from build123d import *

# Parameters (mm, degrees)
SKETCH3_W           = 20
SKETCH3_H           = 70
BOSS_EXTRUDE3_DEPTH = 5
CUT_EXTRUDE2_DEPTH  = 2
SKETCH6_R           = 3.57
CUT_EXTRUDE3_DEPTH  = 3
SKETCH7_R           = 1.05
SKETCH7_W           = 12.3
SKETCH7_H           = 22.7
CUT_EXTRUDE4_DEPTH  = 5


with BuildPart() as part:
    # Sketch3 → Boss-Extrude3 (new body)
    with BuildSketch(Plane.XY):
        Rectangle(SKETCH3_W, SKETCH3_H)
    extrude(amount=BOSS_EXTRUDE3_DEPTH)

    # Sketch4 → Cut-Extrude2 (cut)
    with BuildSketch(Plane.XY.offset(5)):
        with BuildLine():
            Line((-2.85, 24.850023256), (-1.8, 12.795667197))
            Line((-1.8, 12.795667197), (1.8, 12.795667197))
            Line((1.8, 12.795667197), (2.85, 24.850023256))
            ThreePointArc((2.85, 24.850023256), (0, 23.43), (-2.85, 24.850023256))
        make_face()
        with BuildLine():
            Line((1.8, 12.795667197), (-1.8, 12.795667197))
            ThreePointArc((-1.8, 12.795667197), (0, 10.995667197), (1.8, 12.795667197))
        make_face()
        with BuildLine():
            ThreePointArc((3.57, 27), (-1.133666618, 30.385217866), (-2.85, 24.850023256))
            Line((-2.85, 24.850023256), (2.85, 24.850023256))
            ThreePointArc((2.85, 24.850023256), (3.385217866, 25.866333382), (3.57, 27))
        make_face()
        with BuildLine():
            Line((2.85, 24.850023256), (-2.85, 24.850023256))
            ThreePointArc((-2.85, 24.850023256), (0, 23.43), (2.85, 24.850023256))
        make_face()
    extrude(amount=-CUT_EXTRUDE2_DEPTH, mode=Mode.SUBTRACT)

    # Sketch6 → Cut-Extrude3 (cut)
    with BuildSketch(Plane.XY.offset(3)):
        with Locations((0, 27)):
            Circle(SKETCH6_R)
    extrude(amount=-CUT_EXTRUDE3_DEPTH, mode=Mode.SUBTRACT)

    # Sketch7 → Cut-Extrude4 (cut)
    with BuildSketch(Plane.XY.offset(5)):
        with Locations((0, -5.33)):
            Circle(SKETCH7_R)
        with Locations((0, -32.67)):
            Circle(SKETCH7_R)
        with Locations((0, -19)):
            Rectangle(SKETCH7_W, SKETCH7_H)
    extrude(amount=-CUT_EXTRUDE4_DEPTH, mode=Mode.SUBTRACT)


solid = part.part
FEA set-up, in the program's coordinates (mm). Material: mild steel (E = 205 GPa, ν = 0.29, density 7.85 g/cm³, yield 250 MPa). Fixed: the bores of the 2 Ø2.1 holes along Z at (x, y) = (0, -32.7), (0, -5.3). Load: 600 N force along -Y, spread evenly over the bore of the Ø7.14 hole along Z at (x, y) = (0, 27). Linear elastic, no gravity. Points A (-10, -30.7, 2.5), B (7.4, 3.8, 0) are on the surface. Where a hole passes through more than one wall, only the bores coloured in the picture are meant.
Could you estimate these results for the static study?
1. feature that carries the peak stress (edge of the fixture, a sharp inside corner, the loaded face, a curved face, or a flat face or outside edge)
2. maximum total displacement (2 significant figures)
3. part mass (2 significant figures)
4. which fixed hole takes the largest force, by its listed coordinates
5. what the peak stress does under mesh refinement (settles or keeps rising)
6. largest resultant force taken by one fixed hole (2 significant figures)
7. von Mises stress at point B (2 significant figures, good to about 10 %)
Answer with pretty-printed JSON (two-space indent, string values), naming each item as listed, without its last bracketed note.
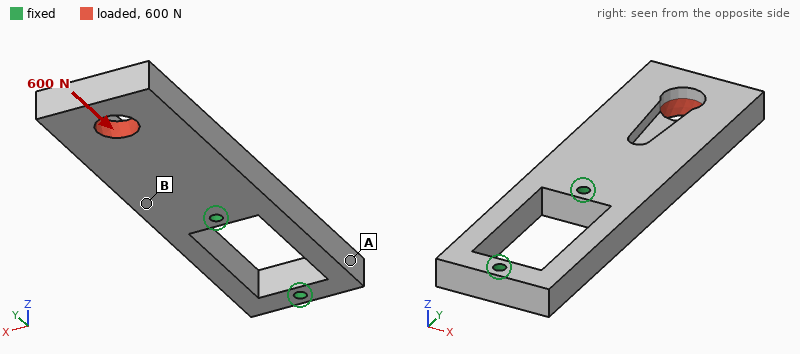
{
  "feature that carries the peak stress": "edge of the fixture",
  "maximum total displacement": "13 µm",
  "part mass": "41 g",
  "which fixed hole takes the largest force, by its listed coordinates": "(0, -5.3)",
  "what the peak stress does under mesh refinement": "keeps rising",
  "largest resultant force taken by one fixed hole": "550 N",
  "von Mises stress at point B": "12 MPa"
}
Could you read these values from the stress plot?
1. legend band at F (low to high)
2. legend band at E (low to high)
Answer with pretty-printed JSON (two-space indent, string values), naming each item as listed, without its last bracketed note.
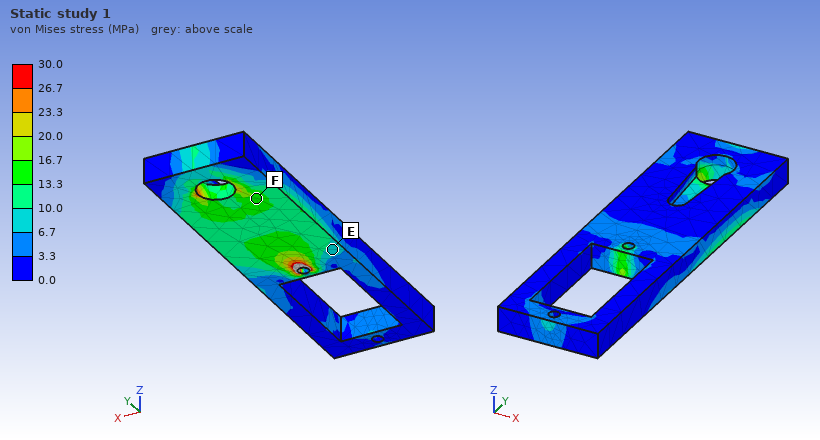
{
  "legend band at F": "13.3 to 16.7 MPa",
  "legend band at E": "6.7 to 10.0 MPa"
}
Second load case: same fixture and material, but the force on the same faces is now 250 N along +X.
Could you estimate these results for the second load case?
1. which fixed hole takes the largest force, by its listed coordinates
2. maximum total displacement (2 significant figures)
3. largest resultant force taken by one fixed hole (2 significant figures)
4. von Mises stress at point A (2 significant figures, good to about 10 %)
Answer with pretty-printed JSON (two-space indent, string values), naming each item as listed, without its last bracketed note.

{
  "which fixed hole takes the largest force, by its listed coordinates": "(0, -5.3)",
  "maximum total displacement": "34 µm",
  "largest resultant force taken by one fixed hole": "340 N",
  "von Mises stress at point A": "22 MPa"
}
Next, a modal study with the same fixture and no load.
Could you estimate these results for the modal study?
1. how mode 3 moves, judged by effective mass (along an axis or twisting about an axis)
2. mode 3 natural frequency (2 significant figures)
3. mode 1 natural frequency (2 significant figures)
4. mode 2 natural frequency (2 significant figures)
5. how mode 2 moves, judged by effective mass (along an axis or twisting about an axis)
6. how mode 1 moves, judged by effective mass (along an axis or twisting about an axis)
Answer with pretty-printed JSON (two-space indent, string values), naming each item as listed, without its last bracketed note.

{
  "how mode 3 moves, judged by effective mass": "twisting about Y",
  "mode 3 natural frequency": "7600 Hz",
  "mode 1 natural frequency": "2400 Hz",
  "mode 2 natural frequency": "4000 Hz",
  "how mode 2 moves, judged by effective mass": "along X",
  "how mode 1 moves, judged by effective mass": "along Z"
}
